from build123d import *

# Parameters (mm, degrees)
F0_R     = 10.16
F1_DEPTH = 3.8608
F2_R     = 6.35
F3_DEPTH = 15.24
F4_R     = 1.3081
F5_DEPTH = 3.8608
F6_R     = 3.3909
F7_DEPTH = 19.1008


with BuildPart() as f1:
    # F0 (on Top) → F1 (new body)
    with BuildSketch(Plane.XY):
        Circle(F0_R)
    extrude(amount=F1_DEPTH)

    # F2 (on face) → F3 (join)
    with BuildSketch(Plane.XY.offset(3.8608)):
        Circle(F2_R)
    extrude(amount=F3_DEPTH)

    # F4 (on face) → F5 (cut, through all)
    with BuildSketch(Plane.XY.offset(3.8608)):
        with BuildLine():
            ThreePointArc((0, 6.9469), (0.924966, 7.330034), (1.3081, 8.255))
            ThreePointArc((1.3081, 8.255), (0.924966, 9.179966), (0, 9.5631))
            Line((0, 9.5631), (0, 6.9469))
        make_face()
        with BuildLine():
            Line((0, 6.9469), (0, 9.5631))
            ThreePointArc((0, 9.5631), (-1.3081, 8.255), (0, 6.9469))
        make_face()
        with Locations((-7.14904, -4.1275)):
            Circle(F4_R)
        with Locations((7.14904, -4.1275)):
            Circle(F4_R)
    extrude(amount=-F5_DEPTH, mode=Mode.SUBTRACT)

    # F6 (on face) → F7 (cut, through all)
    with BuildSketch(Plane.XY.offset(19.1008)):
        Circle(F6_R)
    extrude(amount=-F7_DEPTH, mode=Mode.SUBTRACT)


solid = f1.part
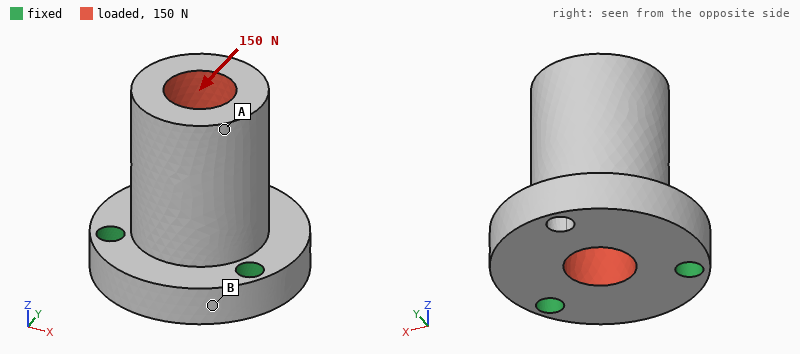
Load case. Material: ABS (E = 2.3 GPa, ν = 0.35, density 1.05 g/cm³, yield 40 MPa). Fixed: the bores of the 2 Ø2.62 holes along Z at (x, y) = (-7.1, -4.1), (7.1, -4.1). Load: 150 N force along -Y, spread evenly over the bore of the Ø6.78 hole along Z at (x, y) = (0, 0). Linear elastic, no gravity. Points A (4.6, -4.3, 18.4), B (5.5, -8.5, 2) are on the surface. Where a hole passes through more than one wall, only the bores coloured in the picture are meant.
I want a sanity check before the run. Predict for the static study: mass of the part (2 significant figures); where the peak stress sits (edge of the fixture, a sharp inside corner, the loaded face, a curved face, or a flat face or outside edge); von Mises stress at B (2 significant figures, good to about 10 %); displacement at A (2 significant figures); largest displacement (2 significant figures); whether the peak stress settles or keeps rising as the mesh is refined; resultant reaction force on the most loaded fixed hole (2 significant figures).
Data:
2.6 g
edge of the fixture
8.6 MPa
0.30 mm
0.36 mm
keeps rising
75 N
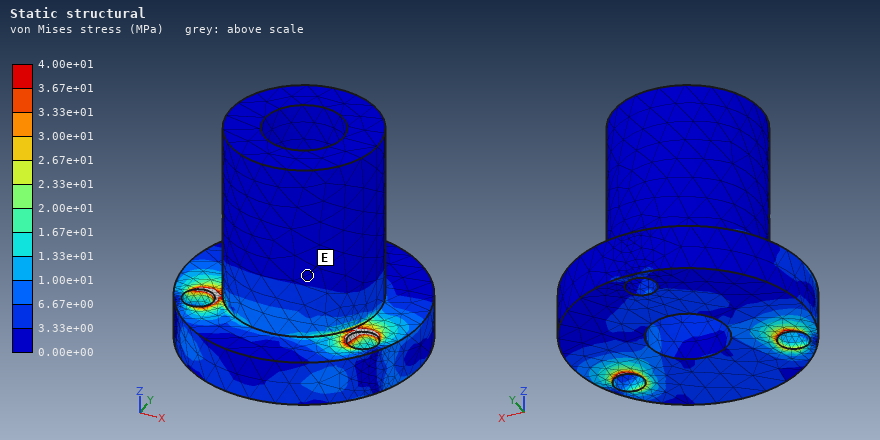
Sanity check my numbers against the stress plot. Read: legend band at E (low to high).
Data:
0.00e+00 to 3.33e+00 MPa
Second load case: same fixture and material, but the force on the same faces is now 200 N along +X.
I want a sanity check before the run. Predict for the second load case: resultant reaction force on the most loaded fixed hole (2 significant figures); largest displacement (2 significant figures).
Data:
160 N
0.12 mm
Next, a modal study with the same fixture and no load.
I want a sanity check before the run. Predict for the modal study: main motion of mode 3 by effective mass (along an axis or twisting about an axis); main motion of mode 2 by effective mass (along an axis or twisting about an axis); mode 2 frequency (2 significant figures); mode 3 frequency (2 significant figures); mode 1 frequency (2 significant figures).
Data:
along X
along X
5500 Hz
10 kHz
2600 Hz
